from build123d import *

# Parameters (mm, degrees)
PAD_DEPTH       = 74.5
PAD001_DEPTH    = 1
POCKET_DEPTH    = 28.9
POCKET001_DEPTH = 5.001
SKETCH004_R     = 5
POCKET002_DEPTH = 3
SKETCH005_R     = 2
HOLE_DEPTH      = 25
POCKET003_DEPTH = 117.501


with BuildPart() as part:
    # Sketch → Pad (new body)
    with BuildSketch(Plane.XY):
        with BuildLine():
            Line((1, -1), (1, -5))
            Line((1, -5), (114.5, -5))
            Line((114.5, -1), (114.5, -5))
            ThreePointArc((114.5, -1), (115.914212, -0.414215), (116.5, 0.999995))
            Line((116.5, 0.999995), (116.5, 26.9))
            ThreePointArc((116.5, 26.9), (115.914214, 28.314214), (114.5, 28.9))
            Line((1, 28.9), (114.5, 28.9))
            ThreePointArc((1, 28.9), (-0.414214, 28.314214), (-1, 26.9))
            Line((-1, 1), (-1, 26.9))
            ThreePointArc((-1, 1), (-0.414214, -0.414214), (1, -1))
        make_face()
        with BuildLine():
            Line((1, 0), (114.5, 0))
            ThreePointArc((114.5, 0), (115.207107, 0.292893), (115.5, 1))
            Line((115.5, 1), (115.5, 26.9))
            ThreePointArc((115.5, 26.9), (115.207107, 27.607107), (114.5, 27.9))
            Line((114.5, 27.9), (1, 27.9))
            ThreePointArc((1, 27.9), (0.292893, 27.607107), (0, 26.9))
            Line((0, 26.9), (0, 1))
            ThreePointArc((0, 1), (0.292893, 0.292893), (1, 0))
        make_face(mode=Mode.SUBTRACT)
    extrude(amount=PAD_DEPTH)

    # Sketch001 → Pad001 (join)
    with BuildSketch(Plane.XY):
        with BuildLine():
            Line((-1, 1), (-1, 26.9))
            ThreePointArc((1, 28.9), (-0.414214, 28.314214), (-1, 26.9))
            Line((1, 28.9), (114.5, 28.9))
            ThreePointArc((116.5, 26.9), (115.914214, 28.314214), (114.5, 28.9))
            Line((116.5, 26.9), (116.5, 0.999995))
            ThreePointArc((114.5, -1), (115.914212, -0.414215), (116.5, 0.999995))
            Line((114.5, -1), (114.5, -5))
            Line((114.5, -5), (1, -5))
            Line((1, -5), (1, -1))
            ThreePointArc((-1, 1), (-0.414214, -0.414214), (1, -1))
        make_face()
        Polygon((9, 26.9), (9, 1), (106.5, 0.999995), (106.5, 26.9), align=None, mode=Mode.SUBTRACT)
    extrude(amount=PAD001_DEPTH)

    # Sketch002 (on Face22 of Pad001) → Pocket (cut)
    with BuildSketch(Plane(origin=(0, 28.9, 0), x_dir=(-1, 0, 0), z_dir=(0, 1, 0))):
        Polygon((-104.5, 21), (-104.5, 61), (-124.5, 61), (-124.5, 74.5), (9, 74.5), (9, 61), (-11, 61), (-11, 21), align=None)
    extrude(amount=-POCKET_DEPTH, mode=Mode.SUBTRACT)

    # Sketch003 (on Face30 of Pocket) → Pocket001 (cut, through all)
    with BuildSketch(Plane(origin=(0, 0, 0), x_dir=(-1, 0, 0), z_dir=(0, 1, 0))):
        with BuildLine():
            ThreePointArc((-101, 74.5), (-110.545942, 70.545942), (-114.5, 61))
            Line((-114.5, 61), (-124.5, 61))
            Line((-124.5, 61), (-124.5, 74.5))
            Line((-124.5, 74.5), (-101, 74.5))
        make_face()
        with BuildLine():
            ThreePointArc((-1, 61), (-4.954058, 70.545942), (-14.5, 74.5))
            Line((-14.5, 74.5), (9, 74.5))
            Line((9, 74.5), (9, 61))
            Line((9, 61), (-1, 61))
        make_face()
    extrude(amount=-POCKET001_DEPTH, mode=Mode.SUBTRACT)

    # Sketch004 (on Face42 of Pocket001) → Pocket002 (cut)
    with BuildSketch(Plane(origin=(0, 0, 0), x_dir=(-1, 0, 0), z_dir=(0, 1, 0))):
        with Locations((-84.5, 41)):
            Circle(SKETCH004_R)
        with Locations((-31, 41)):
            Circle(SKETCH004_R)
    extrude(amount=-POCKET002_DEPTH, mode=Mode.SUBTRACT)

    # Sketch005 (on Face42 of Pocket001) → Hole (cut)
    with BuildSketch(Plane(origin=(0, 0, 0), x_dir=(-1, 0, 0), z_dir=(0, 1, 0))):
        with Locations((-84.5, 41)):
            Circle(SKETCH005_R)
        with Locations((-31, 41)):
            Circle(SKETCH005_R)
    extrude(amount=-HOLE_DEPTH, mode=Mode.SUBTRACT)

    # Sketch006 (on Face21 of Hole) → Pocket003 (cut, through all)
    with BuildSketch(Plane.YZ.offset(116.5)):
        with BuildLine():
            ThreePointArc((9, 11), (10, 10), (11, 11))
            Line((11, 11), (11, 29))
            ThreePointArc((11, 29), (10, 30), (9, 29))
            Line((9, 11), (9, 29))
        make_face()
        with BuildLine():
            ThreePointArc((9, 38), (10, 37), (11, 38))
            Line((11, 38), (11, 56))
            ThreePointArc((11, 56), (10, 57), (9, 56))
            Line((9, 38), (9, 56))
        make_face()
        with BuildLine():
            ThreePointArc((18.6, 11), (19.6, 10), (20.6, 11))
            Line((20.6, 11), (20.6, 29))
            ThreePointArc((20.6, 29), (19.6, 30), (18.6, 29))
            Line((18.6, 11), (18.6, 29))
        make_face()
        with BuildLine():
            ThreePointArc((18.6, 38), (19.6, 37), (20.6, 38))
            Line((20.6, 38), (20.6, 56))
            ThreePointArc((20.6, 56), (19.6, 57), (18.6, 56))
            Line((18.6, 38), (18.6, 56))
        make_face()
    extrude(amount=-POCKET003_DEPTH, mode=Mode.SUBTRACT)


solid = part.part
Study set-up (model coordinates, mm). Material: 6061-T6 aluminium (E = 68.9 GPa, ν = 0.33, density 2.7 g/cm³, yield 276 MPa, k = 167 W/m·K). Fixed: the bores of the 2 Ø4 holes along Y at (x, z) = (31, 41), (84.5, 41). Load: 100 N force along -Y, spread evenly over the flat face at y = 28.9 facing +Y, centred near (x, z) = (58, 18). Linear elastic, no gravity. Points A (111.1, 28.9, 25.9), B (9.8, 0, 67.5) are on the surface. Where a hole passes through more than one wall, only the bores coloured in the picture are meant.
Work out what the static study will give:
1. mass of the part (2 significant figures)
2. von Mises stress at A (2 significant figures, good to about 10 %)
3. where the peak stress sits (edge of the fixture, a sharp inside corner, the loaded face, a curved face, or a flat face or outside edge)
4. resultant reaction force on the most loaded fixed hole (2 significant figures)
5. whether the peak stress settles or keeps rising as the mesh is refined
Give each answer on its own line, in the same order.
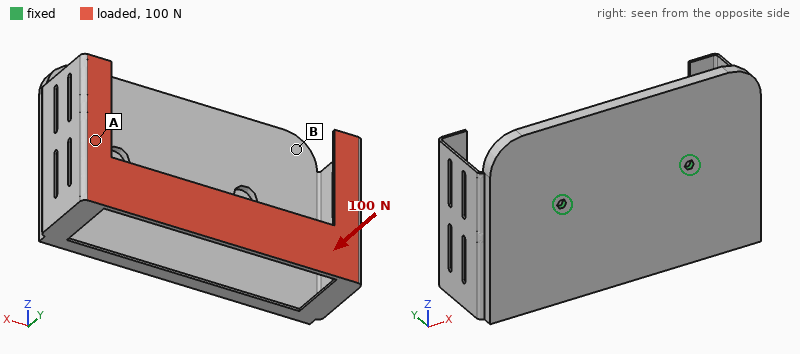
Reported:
130 g
30 MPa
a sharp inside corner
140 N
keeps rising
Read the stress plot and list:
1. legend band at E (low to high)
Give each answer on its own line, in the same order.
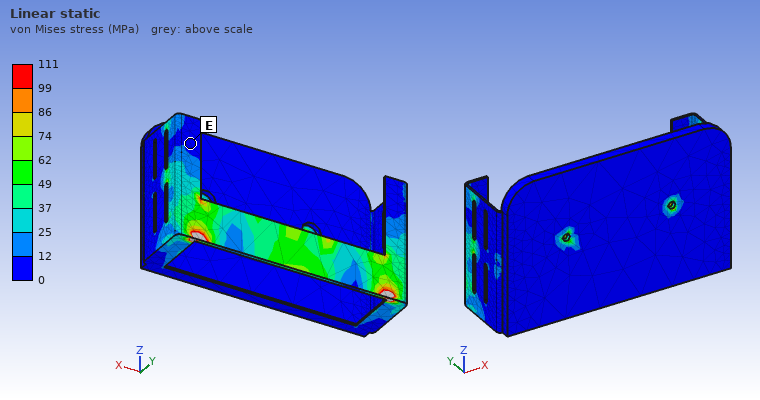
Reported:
0 to 12 MPa
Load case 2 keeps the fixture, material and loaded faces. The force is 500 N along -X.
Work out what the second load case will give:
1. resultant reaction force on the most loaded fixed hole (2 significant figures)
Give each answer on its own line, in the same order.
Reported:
430 N
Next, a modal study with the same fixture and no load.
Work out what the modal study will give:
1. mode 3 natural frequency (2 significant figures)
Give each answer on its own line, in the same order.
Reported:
1000 Hz
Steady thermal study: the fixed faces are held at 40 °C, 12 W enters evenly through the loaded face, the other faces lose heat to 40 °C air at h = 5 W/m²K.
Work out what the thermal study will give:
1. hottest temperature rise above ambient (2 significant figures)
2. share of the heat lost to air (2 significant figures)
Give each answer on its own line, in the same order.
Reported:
61 K
17 %
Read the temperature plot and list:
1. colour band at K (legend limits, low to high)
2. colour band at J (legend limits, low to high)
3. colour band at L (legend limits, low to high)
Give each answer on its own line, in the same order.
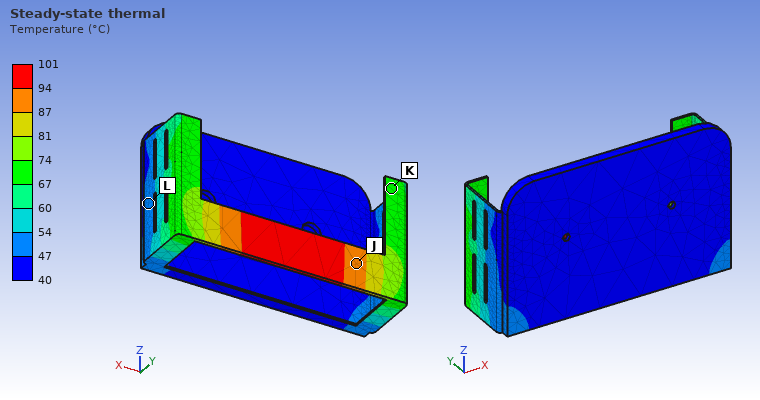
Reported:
67 to 74 °C
87 to 94 °C
47 to 54 °C
